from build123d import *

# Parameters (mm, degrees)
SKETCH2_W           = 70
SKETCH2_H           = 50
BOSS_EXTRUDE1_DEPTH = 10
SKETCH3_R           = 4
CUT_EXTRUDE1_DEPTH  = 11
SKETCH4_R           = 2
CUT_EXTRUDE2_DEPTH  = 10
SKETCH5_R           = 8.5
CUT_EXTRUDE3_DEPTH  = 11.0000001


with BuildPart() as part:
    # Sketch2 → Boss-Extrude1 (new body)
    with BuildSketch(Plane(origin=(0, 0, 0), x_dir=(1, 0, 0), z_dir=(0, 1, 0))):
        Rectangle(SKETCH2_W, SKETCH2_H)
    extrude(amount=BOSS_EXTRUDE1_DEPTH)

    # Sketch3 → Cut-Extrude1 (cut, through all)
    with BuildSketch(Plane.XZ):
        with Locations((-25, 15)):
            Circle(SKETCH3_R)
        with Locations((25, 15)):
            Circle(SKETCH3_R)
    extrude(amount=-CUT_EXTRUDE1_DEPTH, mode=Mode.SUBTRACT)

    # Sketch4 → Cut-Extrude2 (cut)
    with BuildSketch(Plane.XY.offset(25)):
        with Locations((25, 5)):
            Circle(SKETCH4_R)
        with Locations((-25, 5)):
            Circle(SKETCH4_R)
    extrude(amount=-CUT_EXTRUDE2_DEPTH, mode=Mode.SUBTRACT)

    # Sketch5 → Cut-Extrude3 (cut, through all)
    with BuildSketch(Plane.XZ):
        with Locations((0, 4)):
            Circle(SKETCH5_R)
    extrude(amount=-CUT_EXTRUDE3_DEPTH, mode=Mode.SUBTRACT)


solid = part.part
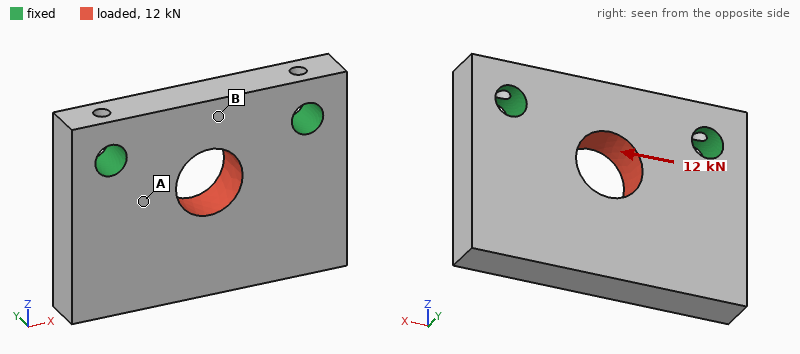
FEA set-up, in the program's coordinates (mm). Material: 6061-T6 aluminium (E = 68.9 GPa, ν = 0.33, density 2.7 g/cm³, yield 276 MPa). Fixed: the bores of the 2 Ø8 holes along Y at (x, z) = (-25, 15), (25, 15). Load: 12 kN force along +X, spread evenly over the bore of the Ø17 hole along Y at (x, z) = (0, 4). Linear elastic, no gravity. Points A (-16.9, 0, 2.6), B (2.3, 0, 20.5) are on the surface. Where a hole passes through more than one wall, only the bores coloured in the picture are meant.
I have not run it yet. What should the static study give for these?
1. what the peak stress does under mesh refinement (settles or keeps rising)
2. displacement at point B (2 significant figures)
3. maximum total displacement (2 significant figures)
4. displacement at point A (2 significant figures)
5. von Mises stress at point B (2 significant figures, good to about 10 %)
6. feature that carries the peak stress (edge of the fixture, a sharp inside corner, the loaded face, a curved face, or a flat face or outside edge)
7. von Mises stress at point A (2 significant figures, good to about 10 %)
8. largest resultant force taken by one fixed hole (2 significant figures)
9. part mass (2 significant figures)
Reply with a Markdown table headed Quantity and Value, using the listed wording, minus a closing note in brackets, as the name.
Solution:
| Quantity | Value |
|---|---|
| what the peak stress does under mesh refinement | keeps rising |
| displacement at point B | 3.8 µm |
| maximum total displacement | 19 µm |
| displacement at point A | 10 µm |
| von Mises stress at point B | 13 MPa |
| feature that carries the peak stress | edge of the fixture |
| von Mises stress at point A | 31 MPa |
| largest resultant force taken by one fixed hole | 6.3 kN |
| part mass | 85 g |
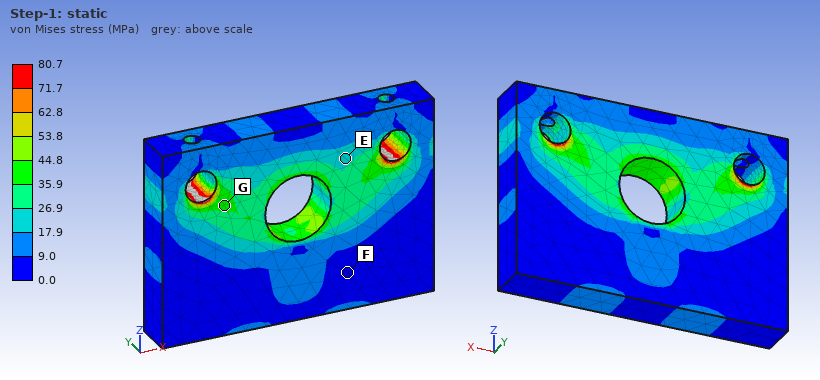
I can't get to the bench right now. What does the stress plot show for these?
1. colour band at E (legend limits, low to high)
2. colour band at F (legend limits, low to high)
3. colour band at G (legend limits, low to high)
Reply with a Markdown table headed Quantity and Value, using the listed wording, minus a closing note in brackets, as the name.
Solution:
| Quantity | Value |
|---|---|
| colour band at E | 17.9 to 26.9 MPa |
| colour band at F | 0.0 to 9.0 MPa |
| colour band at G | 35.9 to 44.8 MPa |
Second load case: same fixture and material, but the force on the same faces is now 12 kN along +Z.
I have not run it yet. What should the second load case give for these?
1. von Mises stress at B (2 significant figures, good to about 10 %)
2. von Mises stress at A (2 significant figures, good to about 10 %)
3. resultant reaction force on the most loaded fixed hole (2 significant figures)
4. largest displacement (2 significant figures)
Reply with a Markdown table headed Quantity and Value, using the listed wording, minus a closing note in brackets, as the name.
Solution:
| Quantity | Value |
|---|---|
| von Mises stress at B | 22 MPa |
| von Mises stress at A | 32 MPa |
| resultant reaction force on the most loaded fixed hole | 6.2 kN |
| largest displacement | 20 µm |
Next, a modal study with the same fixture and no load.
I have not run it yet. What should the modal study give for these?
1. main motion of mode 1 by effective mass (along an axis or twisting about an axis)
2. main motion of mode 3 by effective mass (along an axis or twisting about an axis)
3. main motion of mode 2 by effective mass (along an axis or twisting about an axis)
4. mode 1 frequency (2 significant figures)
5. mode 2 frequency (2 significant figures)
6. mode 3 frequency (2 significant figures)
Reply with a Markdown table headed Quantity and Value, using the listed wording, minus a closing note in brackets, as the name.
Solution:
| Quantity | Value |
|---|---|
| main motion of mode 1 by effective mass | along Y |
| main motion of mode 3 by effective mass | along X |
| main motion of mode 2 by effective mass | twisting about Z |
| mode 1 frequency | 4400 Hz |
| mode 2 frequency | 7800 Hz |
| mode 3 frequency | 13 kHz |
